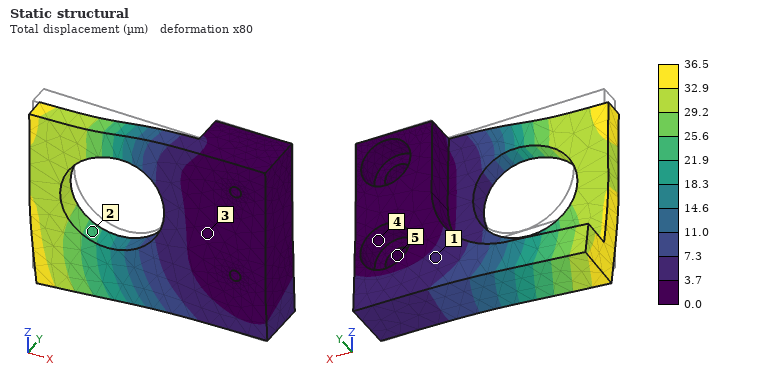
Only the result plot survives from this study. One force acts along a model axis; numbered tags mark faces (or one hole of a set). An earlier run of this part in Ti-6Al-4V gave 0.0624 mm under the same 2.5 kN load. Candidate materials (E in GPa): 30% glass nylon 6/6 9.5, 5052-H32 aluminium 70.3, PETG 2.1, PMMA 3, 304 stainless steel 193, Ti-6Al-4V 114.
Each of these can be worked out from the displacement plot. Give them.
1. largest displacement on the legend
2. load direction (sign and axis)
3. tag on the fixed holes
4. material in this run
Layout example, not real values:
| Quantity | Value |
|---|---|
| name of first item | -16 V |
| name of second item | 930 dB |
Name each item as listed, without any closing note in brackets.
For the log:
| Quantity | Value |
|---|---|
| largest displacement on the legend | 36.5 µm |
| load direction | -Z |
| tag on the fixed holes | 5 |
| material in this run | 304 stainless steel |
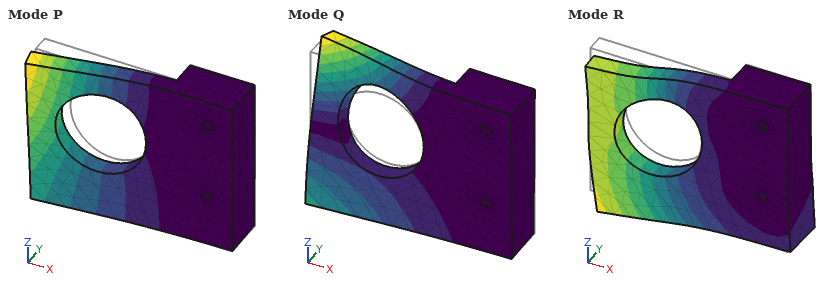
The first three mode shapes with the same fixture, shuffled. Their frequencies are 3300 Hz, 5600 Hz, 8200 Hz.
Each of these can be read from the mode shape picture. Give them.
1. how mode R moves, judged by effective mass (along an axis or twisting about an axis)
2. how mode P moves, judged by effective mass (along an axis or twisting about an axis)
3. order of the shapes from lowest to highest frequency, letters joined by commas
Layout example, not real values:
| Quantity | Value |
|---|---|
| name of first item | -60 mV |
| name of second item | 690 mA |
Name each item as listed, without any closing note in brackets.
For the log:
| Quantity | Value |
|---|---|
| how mode R moves, judged by effective mass | along Z |
| how mode P moves, judged by effective mass | along Y |
| order of the shapes from lowest to highest frequency, letters joined by commas | P, Q, R |
